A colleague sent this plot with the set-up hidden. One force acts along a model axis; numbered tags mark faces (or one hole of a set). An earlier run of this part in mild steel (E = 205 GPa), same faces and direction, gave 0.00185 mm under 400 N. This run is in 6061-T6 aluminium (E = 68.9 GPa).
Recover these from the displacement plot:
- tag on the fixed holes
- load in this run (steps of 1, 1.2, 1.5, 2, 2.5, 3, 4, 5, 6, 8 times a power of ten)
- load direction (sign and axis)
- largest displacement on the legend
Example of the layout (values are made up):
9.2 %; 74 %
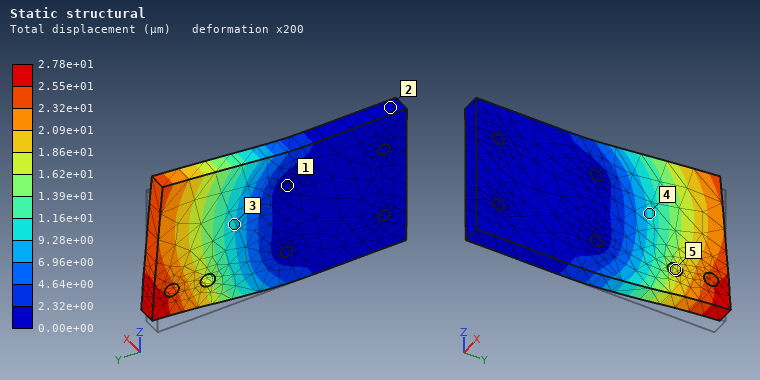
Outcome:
1; 2 kN; +Z; 2.78e+01 µm
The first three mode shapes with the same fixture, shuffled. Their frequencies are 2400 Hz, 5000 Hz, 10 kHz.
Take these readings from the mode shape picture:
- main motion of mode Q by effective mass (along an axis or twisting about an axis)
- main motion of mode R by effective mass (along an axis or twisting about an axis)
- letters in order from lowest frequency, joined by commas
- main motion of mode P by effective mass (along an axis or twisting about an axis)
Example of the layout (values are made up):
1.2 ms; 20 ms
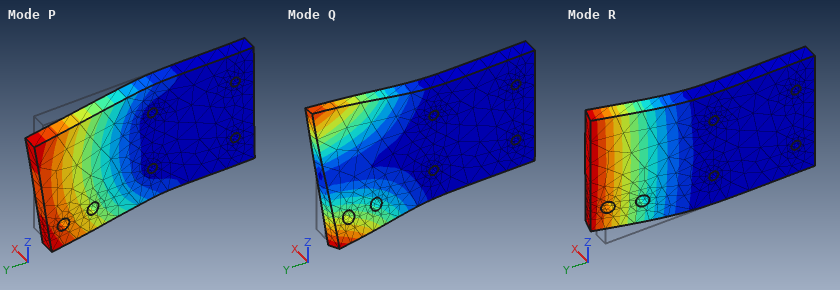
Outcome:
twisting about Y; along X; R, Q, P; along Z
